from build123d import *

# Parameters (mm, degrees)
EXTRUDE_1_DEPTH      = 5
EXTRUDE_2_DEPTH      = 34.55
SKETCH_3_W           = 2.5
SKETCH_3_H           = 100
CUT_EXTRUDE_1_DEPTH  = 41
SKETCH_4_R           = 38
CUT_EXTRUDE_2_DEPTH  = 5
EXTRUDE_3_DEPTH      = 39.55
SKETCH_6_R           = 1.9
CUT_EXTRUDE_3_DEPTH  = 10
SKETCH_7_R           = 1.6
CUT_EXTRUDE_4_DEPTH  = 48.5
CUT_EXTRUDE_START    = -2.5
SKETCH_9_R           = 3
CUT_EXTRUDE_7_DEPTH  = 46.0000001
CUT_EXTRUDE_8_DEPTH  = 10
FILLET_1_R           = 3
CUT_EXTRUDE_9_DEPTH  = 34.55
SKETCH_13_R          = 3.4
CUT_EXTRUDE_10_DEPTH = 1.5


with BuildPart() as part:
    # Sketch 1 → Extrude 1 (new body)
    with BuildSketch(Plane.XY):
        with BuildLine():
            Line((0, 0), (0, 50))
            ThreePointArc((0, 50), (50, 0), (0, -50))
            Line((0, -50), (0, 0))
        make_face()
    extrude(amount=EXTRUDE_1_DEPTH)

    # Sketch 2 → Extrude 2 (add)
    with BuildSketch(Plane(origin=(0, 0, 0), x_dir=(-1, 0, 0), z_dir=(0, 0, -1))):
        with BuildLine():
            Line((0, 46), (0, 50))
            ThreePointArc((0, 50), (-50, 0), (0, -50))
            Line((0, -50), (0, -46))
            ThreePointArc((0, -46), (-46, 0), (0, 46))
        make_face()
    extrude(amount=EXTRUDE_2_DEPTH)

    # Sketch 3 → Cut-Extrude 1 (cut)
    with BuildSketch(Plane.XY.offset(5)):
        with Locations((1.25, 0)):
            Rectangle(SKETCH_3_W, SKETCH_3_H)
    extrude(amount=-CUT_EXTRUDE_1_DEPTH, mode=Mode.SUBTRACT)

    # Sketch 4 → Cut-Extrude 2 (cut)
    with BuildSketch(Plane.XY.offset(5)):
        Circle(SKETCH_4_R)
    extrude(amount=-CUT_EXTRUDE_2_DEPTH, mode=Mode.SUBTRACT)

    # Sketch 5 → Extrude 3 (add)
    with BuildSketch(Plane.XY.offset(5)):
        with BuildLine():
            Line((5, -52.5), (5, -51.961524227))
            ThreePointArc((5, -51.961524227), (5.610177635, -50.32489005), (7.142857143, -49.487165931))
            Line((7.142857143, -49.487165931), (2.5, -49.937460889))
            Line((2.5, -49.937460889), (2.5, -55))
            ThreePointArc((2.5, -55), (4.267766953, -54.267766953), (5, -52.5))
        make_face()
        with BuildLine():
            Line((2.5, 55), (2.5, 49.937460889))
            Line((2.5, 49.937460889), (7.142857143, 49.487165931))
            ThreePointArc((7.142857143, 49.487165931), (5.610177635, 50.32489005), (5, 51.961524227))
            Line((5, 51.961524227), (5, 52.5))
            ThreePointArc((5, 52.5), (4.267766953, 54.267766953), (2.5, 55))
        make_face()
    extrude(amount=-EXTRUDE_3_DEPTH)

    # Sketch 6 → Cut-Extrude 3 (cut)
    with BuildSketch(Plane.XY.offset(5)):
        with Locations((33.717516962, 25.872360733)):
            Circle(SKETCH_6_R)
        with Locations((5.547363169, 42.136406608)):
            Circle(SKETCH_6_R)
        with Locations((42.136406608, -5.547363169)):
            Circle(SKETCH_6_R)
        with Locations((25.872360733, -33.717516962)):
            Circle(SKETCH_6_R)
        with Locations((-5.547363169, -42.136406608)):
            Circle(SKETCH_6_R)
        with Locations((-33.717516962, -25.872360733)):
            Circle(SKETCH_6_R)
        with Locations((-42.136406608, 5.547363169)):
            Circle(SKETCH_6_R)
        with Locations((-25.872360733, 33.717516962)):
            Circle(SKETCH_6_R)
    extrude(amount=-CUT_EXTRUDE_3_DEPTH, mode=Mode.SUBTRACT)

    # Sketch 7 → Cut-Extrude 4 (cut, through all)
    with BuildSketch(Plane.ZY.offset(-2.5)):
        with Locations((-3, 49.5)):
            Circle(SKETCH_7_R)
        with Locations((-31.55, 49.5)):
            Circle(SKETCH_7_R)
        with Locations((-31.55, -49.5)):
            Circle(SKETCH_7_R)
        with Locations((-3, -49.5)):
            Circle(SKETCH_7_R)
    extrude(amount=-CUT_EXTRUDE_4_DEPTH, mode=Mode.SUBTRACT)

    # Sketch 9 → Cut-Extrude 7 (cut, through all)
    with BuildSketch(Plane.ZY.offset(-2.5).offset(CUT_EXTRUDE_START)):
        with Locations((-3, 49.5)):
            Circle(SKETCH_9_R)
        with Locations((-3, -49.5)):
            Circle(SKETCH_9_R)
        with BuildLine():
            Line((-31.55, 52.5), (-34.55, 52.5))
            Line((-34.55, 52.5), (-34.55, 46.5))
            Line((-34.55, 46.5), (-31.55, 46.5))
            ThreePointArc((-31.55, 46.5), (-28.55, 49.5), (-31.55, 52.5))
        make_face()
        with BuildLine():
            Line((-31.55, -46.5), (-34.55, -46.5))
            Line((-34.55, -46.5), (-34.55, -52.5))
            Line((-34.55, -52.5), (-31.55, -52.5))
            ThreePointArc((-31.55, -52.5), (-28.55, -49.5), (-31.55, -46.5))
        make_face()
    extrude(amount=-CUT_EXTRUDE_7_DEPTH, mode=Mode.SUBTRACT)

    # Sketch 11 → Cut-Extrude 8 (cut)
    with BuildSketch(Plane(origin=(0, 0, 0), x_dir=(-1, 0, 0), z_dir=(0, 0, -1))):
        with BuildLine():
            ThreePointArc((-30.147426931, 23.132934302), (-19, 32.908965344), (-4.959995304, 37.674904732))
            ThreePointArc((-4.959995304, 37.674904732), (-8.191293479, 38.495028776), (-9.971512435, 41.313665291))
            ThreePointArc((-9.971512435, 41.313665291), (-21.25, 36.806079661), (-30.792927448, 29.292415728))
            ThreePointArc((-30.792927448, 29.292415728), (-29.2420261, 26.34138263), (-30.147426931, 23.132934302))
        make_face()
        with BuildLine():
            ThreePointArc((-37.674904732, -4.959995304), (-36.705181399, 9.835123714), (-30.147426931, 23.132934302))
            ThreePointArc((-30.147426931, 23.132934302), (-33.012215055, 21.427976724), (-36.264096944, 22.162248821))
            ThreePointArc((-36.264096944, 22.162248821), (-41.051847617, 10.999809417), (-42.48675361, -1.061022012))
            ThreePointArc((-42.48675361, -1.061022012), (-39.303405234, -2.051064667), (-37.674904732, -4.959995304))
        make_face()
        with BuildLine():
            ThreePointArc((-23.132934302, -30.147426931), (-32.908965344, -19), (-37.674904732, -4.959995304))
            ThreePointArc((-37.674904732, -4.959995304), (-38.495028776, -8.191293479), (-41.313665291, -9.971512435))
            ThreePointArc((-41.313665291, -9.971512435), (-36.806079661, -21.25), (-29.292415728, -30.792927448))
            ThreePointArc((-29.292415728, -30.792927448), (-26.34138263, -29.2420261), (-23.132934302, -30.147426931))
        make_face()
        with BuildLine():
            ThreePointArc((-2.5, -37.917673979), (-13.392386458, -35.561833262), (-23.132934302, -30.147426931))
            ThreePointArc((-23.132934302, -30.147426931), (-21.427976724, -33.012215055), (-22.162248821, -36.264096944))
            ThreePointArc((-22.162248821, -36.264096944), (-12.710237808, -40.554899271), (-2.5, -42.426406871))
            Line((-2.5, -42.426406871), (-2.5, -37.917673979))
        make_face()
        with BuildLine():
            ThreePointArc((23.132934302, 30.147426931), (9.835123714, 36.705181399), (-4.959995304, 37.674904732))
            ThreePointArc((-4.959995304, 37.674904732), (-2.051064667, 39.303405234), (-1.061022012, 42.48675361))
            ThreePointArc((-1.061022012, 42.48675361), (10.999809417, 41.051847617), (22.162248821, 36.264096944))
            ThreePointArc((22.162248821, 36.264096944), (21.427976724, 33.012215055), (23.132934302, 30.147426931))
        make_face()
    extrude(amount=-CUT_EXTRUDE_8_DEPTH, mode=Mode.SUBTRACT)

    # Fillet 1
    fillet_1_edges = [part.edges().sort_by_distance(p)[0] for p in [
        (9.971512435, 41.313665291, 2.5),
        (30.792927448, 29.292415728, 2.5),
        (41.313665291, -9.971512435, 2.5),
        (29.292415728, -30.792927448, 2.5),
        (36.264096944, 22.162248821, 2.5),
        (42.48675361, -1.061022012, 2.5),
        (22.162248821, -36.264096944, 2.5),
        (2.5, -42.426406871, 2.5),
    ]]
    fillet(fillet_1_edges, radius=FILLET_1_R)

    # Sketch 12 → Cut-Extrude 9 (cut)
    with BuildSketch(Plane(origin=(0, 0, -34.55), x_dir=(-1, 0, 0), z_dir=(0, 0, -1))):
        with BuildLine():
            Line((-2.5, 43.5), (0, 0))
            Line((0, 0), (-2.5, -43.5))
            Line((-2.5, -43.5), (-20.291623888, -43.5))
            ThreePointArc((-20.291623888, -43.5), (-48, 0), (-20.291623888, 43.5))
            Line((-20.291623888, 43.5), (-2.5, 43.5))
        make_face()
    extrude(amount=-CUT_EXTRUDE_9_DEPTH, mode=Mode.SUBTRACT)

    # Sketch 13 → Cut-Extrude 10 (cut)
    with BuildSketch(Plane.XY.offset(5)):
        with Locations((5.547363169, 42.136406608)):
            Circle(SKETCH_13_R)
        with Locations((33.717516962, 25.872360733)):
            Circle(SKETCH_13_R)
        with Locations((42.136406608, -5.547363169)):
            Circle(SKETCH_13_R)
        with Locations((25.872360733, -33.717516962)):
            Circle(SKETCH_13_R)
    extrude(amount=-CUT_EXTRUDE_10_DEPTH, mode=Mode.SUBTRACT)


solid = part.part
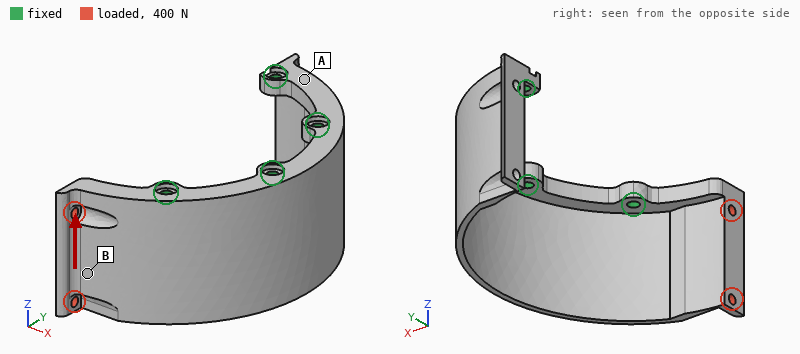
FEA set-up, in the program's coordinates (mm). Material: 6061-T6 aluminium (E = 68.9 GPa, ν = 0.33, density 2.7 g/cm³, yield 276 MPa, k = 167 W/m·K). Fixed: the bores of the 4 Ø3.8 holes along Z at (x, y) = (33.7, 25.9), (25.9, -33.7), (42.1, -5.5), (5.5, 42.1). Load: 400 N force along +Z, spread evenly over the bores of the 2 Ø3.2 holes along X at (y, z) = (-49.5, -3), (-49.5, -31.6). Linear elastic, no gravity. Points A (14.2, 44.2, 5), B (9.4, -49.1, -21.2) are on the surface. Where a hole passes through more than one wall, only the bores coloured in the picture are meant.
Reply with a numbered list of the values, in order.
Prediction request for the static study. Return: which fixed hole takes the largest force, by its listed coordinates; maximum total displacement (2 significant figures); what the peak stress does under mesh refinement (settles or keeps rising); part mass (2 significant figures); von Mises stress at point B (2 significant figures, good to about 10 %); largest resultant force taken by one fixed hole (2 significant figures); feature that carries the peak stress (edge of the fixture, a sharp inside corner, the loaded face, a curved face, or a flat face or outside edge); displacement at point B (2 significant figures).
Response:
1. (25.9, -33.7)
2. 0.20 mm
3. keeps rising
4. 50 g
5. 17 MPa
6. 670 N
7. edge of the fixture
8. 0.12 mm
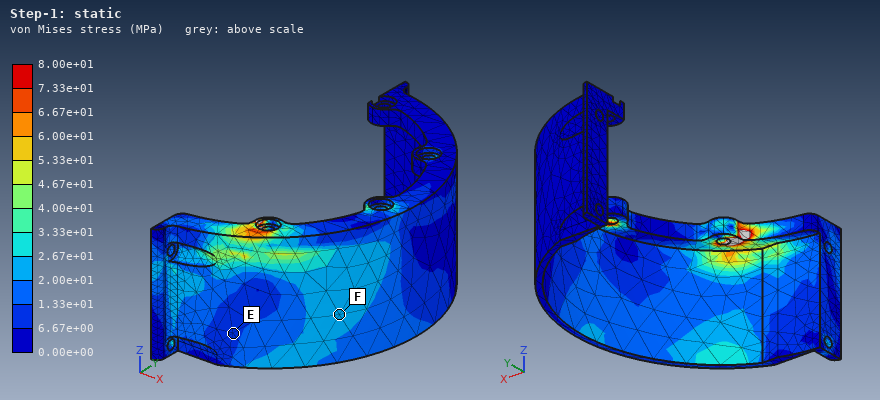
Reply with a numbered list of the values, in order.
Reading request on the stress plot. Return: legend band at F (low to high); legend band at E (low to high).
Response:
1. 2.00e+01 to 2.67e+01 MPa
2. 6.67e+00 to 1.33e+01 MPa
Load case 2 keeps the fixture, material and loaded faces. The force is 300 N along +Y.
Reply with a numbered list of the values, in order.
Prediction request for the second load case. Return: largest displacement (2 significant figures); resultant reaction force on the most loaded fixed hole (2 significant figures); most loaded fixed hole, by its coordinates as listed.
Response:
1. 0.62 mm
2. 580 N
3. (25.9, -33.7)
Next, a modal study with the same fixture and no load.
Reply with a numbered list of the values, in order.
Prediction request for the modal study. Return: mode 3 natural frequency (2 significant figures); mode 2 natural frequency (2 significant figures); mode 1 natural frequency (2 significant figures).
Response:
1. 2600 Hz
2. 2500 Hz
3. 1700 Hz
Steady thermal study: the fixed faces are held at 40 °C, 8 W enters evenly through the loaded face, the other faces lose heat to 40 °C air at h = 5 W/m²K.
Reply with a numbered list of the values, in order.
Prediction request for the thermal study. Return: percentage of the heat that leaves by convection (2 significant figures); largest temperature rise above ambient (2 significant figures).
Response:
1. 3.4 %
2. 23 K
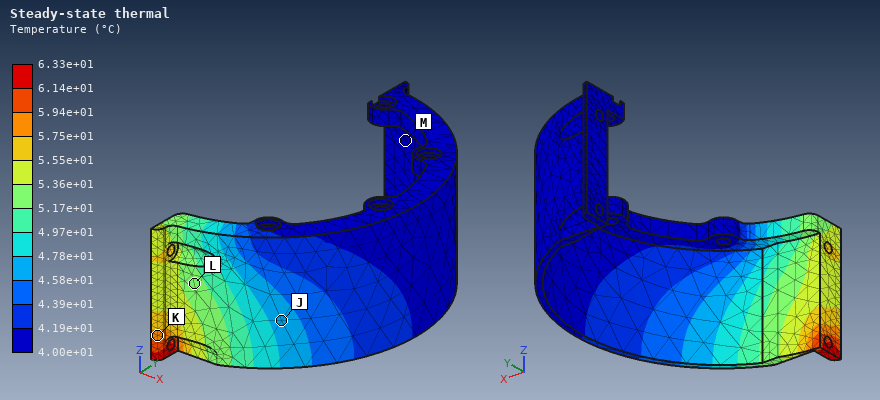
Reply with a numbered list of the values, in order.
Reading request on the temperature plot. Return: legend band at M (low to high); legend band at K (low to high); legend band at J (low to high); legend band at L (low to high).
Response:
1. 4.00e+01 to 4.19e+01 °C
2. 5.75e+01 to 5.94e+01 °C
3. 4.58e+01 to 4.78e+01 °C
4. 5.17e+01 to 5.36e+01 °C
